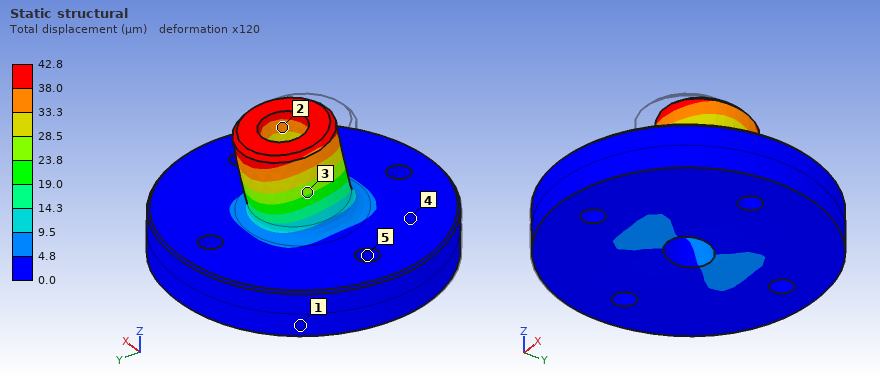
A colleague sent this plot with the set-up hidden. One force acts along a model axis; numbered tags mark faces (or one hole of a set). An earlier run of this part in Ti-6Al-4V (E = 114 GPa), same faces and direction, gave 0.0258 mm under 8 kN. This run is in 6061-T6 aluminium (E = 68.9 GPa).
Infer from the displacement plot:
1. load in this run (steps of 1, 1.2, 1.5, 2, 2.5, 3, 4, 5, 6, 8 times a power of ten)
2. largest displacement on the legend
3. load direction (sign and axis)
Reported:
8 kN
42.8 µm
+Y
